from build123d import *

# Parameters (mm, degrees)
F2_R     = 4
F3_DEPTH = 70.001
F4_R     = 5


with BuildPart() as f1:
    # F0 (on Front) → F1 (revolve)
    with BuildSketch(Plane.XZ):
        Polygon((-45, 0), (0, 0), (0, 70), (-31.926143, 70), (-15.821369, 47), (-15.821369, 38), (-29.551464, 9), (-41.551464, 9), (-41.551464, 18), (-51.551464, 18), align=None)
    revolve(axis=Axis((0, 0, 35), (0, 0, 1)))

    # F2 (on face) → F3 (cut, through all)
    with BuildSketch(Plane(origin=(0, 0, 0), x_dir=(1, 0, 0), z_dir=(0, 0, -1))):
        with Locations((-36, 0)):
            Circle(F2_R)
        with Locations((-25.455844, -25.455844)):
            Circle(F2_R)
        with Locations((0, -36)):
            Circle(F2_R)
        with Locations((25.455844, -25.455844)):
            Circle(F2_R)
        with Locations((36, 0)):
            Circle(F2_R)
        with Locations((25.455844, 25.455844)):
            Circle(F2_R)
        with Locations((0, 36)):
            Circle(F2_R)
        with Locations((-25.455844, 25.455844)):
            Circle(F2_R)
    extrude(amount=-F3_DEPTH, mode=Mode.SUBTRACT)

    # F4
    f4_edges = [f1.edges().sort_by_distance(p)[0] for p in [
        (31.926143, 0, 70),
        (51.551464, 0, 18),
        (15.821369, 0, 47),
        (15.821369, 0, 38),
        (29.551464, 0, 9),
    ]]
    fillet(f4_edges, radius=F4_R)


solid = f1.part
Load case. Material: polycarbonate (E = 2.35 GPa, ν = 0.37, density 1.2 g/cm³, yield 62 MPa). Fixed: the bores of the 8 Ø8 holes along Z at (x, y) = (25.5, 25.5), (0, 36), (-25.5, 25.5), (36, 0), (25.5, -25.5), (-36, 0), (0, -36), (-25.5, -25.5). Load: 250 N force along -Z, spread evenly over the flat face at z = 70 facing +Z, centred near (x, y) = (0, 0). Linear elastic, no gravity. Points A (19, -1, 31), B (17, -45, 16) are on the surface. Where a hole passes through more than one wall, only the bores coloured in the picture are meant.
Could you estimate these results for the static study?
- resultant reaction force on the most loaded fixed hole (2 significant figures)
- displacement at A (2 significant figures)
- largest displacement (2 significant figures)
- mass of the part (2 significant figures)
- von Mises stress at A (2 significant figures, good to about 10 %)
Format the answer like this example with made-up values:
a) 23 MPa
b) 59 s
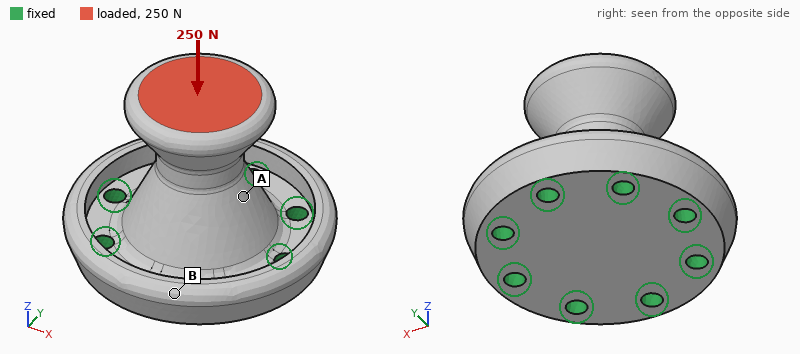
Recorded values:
a) 38 N
b) 4.0 µm
c) 8.4 µm
d) 200 g
e) 0.21 MPa
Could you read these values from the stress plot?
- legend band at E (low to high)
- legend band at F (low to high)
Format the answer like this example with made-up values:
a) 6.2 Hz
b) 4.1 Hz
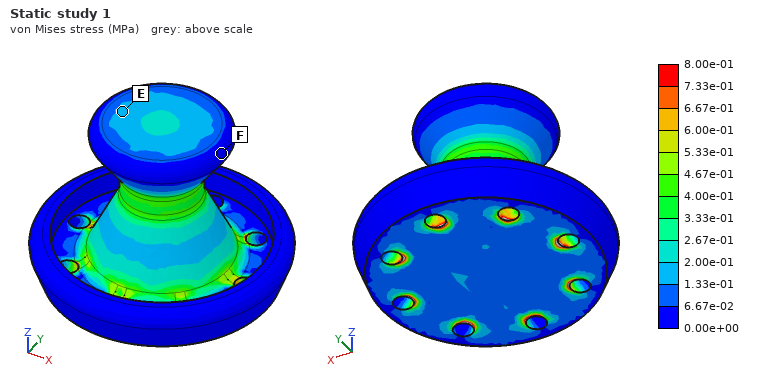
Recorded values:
a) 1.33e-01 to 2.00e-01 MPa
b) 0.00e+00 to 6.67e-02 MPa
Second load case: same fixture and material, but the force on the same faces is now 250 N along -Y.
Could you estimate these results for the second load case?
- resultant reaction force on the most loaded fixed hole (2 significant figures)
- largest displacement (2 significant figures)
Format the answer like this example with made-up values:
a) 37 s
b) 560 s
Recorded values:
a) 150 N
b) 0.11 mm
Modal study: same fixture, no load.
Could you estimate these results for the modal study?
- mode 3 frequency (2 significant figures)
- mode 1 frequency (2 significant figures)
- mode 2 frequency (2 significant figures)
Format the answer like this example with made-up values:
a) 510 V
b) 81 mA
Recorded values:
a) 2400 Hz
b) 1400 Hz
c) 1400 Hz
